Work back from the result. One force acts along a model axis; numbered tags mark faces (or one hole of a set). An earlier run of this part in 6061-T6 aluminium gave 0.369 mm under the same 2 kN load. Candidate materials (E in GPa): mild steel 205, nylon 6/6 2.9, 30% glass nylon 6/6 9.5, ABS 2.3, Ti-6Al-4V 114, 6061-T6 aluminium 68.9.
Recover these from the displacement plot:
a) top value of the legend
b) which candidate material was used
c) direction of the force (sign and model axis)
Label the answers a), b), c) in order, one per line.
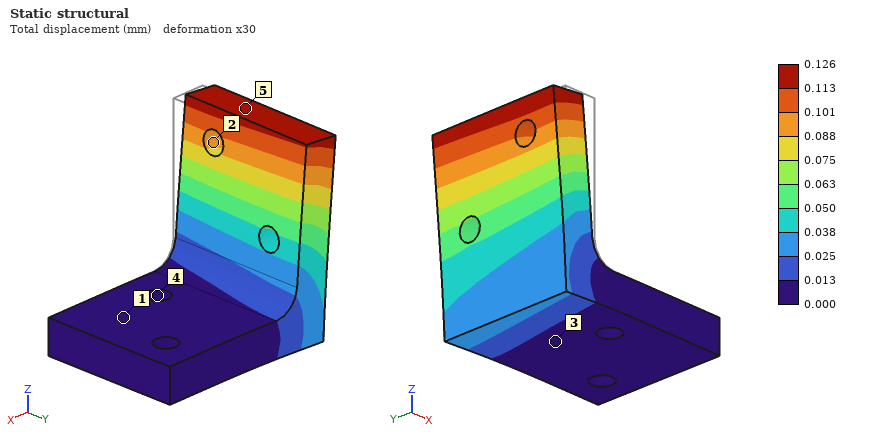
a) 0.126 mm
b) mild steel
c) -X
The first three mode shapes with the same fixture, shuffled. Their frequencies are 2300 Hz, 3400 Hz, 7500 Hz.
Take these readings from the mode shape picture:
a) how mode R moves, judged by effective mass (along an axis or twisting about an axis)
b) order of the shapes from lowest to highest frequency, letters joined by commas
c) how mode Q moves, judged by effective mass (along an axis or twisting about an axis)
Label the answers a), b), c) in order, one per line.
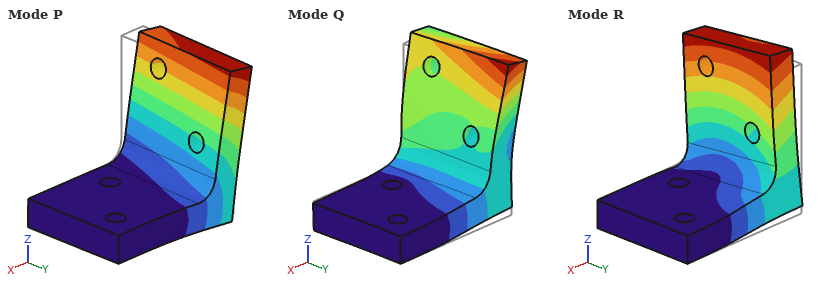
a) along Y
b) P, R, Q
c) along Z
